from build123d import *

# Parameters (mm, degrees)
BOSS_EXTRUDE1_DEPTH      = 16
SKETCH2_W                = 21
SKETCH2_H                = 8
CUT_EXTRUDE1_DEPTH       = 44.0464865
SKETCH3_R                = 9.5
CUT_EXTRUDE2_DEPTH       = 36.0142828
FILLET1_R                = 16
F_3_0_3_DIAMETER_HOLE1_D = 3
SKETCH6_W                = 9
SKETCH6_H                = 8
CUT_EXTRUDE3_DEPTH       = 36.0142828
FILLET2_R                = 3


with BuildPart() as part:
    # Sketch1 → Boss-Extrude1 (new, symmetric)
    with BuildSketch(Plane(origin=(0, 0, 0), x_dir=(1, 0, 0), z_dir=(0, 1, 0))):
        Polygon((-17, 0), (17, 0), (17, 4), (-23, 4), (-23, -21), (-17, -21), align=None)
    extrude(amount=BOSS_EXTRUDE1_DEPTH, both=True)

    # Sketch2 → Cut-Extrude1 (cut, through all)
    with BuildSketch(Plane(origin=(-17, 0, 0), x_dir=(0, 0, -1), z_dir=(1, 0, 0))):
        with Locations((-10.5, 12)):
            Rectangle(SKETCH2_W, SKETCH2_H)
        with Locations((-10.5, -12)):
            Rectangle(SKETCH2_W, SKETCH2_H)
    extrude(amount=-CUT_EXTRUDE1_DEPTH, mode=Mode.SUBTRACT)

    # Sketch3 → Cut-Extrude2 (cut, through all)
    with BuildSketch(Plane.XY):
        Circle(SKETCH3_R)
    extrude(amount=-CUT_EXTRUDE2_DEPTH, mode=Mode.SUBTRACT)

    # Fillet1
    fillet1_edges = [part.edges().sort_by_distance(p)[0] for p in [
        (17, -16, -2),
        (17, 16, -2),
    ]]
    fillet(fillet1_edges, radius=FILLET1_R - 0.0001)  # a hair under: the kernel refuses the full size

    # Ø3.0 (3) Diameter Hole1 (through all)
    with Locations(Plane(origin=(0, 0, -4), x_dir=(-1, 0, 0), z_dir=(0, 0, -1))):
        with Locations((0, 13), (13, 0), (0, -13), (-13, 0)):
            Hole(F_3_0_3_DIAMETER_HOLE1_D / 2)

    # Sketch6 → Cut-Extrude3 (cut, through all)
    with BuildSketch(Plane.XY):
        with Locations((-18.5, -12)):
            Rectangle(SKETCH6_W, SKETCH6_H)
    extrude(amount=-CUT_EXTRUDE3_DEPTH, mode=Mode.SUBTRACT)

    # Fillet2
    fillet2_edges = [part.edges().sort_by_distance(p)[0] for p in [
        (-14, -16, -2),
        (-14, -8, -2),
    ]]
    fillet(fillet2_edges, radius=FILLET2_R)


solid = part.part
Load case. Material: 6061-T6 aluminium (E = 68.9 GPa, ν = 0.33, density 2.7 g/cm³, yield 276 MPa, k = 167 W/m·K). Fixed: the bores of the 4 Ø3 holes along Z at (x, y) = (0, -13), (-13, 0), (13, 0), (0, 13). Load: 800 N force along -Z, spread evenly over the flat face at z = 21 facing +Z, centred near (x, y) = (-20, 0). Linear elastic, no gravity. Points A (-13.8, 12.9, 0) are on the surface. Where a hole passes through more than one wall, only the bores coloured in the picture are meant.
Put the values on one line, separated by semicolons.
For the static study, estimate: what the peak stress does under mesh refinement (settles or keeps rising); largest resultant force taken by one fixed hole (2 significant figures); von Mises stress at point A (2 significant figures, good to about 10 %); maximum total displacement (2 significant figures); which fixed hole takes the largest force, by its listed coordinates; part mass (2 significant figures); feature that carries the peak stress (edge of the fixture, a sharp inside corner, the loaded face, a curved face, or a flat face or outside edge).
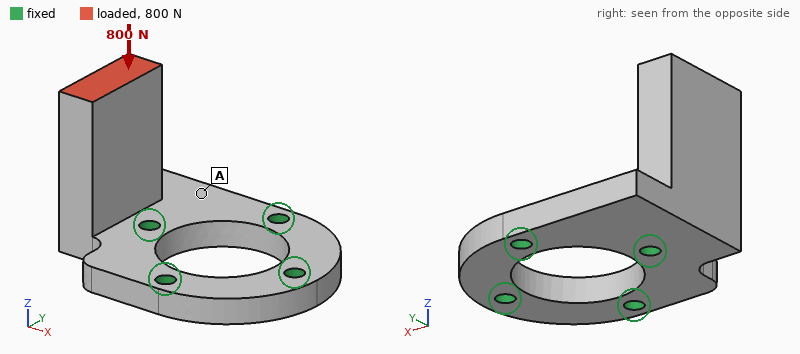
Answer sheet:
keeps rising; 890 N; 21 MPa; 77 µm; (-13, 0); 14 g; edge of the fixture
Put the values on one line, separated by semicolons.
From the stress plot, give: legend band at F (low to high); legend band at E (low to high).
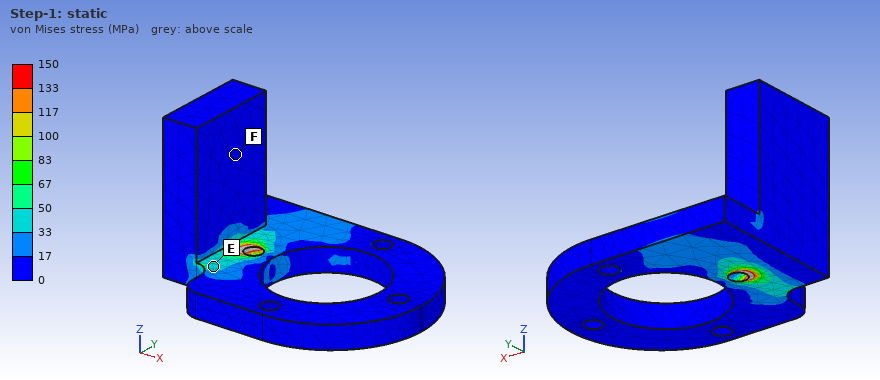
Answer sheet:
0 to 17 MPa; 33 to 50 MPa
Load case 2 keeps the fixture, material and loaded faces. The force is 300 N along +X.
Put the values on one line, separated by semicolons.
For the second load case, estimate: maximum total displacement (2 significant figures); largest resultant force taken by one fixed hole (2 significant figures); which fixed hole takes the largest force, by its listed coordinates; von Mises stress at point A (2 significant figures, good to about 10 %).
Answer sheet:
0.19 mm; 320 N; (-13, 0); 43 MPa
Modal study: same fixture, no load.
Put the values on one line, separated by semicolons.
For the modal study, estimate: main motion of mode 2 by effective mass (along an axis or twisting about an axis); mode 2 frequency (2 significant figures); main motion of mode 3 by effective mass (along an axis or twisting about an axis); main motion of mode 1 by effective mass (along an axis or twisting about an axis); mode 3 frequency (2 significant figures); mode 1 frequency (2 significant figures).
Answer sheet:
along Y; 6100 Hz; along Z; along X; 17 kHz; 4500 Hz
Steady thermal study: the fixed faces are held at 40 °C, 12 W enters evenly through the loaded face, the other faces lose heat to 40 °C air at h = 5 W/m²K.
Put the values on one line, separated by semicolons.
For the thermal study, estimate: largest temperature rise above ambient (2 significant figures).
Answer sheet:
23 K
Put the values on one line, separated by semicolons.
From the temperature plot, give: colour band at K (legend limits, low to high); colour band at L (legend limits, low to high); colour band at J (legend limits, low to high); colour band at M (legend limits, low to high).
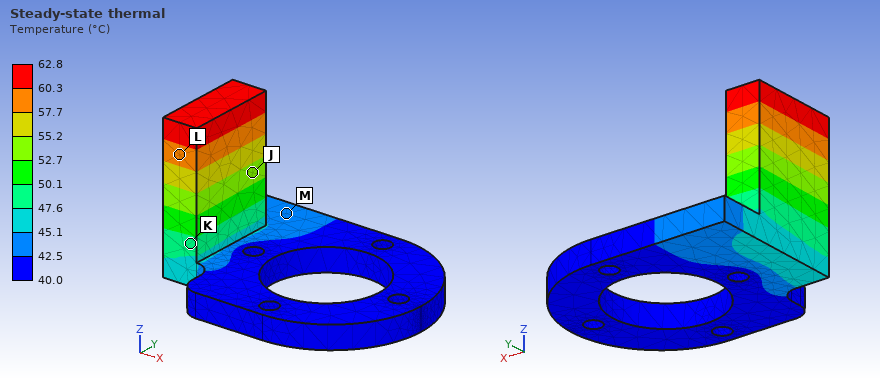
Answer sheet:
47.6 to 50.1 °C; 57.7 to 60.3 °C; 52.7 to 55.2 °C; 42.5 to 45.1 °C
